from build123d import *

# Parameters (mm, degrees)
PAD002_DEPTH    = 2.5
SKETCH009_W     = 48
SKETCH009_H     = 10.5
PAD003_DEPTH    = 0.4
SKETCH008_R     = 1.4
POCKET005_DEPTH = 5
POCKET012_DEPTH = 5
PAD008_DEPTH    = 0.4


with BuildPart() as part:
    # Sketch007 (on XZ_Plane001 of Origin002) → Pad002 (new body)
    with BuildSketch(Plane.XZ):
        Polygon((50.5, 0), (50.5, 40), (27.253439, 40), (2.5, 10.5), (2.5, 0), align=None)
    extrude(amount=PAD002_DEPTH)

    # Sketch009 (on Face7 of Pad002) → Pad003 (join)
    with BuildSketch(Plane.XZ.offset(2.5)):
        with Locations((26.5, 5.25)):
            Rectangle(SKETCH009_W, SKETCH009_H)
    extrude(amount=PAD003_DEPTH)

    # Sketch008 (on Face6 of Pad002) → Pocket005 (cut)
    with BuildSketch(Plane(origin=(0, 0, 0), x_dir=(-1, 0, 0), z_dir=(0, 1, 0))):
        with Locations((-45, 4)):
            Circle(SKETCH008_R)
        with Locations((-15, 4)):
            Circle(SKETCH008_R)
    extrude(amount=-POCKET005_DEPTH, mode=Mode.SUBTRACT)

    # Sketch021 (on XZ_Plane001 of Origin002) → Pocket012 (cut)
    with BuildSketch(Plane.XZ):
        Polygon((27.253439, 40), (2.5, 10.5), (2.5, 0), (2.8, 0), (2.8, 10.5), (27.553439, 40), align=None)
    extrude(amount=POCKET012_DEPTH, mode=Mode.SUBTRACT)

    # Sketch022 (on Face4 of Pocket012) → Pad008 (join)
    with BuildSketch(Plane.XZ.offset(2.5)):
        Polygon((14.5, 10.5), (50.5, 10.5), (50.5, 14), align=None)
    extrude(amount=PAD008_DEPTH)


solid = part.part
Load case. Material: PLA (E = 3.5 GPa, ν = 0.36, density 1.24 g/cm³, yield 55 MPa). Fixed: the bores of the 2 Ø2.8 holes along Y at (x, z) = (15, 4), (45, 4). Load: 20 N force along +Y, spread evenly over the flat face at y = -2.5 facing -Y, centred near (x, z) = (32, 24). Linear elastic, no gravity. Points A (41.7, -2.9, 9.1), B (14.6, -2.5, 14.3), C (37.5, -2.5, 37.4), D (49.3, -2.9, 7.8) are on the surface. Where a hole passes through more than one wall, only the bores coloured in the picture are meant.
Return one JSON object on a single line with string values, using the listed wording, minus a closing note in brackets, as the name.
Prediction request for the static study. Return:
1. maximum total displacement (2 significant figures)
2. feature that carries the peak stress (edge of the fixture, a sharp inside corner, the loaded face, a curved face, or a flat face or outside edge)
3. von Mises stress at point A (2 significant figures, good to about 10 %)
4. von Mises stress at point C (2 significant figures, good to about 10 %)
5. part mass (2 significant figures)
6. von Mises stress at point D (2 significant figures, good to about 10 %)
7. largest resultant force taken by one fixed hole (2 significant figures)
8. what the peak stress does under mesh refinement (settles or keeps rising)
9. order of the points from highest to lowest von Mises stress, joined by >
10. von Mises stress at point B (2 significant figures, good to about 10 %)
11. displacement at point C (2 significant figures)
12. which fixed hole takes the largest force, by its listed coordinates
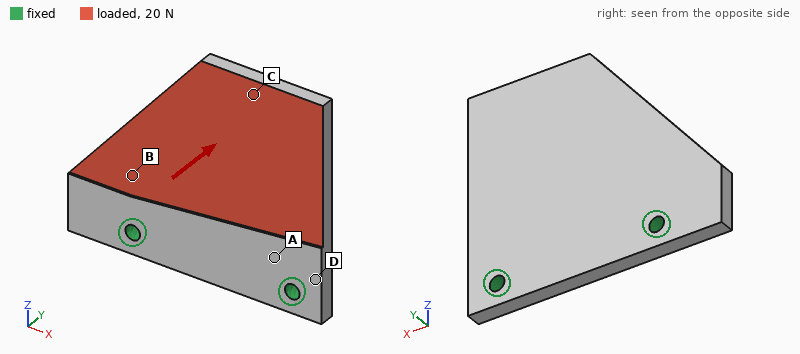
{"maximum total displacement": "0.68 mm", "feature that carries the peak stress": "edge of the fixture", "von Mises stress at point A": "5.9 MPa", "von Mises stress at point C": "1.1 MPa", "part mass": "5.0 g", "von Mises stress at point D": "7.6 MPa", "largest resultant force taken by one fixed hole": "11 N", "what the peak stress does under mesh refinement": "keeps rising", "order of the points from highest to lowest von Mises stress, joined by >": "D > A > B > C", "von Mises stress at point B": "4.0 MPa", "displacement at point C": "0.61 mm", "which fixed hole takes the largest force, by its listed coordinates": "(45, 4)"}
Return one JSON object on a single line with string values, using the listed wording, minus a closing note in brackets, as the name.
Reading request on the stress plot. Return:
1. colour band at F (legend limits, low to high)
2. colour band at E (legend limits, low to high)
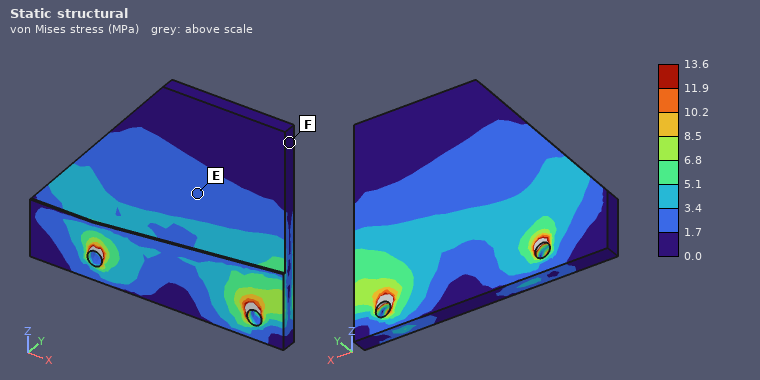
{"colour band at F": "0.0 to 1.7 MPa", "colour band at E": "1.7 to 3.4 MPa"}
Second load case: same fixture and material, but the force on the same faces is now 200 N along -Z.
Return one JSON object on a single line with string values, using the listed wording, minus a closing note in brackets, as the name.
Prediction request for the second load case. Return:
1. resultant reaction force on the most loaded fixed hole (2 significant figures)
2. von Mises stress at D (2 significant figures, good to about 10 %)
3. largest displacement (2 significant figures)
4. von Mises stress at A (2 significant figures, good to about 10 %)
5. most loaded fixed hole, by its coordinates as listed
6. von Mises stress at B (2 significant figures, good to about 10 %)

{"resultant reaction force on the most loaded fixed hole": "110 N", "von Mises stress at D": "5.9 MPa", "largest displacement": "0.57 mm", "von Mises stress at A": "6.8 MPa", "most loaded fixed hole, by its coordinates as listed": "(45, 4)", "von Mises stress at B": "5.7 MPa"}
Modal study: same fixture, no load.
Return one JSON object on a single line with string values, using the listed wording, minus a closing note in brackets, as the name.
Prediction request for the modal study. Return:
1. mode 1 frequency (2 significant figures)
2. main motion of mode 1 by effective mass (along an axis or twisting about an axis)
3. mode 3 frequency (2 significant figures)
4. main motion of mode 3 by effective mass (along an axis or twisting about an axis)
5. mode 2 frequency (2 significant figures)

{"mode 1 frequency": "640 Hz", "main motion of mode 1 by effective mass": "along Y", "mode 3 frequency": "3200 Hz", "main motion of mode 3 by effective mass": "along Y", "mode 2 frequency": "1800 Hz"}
